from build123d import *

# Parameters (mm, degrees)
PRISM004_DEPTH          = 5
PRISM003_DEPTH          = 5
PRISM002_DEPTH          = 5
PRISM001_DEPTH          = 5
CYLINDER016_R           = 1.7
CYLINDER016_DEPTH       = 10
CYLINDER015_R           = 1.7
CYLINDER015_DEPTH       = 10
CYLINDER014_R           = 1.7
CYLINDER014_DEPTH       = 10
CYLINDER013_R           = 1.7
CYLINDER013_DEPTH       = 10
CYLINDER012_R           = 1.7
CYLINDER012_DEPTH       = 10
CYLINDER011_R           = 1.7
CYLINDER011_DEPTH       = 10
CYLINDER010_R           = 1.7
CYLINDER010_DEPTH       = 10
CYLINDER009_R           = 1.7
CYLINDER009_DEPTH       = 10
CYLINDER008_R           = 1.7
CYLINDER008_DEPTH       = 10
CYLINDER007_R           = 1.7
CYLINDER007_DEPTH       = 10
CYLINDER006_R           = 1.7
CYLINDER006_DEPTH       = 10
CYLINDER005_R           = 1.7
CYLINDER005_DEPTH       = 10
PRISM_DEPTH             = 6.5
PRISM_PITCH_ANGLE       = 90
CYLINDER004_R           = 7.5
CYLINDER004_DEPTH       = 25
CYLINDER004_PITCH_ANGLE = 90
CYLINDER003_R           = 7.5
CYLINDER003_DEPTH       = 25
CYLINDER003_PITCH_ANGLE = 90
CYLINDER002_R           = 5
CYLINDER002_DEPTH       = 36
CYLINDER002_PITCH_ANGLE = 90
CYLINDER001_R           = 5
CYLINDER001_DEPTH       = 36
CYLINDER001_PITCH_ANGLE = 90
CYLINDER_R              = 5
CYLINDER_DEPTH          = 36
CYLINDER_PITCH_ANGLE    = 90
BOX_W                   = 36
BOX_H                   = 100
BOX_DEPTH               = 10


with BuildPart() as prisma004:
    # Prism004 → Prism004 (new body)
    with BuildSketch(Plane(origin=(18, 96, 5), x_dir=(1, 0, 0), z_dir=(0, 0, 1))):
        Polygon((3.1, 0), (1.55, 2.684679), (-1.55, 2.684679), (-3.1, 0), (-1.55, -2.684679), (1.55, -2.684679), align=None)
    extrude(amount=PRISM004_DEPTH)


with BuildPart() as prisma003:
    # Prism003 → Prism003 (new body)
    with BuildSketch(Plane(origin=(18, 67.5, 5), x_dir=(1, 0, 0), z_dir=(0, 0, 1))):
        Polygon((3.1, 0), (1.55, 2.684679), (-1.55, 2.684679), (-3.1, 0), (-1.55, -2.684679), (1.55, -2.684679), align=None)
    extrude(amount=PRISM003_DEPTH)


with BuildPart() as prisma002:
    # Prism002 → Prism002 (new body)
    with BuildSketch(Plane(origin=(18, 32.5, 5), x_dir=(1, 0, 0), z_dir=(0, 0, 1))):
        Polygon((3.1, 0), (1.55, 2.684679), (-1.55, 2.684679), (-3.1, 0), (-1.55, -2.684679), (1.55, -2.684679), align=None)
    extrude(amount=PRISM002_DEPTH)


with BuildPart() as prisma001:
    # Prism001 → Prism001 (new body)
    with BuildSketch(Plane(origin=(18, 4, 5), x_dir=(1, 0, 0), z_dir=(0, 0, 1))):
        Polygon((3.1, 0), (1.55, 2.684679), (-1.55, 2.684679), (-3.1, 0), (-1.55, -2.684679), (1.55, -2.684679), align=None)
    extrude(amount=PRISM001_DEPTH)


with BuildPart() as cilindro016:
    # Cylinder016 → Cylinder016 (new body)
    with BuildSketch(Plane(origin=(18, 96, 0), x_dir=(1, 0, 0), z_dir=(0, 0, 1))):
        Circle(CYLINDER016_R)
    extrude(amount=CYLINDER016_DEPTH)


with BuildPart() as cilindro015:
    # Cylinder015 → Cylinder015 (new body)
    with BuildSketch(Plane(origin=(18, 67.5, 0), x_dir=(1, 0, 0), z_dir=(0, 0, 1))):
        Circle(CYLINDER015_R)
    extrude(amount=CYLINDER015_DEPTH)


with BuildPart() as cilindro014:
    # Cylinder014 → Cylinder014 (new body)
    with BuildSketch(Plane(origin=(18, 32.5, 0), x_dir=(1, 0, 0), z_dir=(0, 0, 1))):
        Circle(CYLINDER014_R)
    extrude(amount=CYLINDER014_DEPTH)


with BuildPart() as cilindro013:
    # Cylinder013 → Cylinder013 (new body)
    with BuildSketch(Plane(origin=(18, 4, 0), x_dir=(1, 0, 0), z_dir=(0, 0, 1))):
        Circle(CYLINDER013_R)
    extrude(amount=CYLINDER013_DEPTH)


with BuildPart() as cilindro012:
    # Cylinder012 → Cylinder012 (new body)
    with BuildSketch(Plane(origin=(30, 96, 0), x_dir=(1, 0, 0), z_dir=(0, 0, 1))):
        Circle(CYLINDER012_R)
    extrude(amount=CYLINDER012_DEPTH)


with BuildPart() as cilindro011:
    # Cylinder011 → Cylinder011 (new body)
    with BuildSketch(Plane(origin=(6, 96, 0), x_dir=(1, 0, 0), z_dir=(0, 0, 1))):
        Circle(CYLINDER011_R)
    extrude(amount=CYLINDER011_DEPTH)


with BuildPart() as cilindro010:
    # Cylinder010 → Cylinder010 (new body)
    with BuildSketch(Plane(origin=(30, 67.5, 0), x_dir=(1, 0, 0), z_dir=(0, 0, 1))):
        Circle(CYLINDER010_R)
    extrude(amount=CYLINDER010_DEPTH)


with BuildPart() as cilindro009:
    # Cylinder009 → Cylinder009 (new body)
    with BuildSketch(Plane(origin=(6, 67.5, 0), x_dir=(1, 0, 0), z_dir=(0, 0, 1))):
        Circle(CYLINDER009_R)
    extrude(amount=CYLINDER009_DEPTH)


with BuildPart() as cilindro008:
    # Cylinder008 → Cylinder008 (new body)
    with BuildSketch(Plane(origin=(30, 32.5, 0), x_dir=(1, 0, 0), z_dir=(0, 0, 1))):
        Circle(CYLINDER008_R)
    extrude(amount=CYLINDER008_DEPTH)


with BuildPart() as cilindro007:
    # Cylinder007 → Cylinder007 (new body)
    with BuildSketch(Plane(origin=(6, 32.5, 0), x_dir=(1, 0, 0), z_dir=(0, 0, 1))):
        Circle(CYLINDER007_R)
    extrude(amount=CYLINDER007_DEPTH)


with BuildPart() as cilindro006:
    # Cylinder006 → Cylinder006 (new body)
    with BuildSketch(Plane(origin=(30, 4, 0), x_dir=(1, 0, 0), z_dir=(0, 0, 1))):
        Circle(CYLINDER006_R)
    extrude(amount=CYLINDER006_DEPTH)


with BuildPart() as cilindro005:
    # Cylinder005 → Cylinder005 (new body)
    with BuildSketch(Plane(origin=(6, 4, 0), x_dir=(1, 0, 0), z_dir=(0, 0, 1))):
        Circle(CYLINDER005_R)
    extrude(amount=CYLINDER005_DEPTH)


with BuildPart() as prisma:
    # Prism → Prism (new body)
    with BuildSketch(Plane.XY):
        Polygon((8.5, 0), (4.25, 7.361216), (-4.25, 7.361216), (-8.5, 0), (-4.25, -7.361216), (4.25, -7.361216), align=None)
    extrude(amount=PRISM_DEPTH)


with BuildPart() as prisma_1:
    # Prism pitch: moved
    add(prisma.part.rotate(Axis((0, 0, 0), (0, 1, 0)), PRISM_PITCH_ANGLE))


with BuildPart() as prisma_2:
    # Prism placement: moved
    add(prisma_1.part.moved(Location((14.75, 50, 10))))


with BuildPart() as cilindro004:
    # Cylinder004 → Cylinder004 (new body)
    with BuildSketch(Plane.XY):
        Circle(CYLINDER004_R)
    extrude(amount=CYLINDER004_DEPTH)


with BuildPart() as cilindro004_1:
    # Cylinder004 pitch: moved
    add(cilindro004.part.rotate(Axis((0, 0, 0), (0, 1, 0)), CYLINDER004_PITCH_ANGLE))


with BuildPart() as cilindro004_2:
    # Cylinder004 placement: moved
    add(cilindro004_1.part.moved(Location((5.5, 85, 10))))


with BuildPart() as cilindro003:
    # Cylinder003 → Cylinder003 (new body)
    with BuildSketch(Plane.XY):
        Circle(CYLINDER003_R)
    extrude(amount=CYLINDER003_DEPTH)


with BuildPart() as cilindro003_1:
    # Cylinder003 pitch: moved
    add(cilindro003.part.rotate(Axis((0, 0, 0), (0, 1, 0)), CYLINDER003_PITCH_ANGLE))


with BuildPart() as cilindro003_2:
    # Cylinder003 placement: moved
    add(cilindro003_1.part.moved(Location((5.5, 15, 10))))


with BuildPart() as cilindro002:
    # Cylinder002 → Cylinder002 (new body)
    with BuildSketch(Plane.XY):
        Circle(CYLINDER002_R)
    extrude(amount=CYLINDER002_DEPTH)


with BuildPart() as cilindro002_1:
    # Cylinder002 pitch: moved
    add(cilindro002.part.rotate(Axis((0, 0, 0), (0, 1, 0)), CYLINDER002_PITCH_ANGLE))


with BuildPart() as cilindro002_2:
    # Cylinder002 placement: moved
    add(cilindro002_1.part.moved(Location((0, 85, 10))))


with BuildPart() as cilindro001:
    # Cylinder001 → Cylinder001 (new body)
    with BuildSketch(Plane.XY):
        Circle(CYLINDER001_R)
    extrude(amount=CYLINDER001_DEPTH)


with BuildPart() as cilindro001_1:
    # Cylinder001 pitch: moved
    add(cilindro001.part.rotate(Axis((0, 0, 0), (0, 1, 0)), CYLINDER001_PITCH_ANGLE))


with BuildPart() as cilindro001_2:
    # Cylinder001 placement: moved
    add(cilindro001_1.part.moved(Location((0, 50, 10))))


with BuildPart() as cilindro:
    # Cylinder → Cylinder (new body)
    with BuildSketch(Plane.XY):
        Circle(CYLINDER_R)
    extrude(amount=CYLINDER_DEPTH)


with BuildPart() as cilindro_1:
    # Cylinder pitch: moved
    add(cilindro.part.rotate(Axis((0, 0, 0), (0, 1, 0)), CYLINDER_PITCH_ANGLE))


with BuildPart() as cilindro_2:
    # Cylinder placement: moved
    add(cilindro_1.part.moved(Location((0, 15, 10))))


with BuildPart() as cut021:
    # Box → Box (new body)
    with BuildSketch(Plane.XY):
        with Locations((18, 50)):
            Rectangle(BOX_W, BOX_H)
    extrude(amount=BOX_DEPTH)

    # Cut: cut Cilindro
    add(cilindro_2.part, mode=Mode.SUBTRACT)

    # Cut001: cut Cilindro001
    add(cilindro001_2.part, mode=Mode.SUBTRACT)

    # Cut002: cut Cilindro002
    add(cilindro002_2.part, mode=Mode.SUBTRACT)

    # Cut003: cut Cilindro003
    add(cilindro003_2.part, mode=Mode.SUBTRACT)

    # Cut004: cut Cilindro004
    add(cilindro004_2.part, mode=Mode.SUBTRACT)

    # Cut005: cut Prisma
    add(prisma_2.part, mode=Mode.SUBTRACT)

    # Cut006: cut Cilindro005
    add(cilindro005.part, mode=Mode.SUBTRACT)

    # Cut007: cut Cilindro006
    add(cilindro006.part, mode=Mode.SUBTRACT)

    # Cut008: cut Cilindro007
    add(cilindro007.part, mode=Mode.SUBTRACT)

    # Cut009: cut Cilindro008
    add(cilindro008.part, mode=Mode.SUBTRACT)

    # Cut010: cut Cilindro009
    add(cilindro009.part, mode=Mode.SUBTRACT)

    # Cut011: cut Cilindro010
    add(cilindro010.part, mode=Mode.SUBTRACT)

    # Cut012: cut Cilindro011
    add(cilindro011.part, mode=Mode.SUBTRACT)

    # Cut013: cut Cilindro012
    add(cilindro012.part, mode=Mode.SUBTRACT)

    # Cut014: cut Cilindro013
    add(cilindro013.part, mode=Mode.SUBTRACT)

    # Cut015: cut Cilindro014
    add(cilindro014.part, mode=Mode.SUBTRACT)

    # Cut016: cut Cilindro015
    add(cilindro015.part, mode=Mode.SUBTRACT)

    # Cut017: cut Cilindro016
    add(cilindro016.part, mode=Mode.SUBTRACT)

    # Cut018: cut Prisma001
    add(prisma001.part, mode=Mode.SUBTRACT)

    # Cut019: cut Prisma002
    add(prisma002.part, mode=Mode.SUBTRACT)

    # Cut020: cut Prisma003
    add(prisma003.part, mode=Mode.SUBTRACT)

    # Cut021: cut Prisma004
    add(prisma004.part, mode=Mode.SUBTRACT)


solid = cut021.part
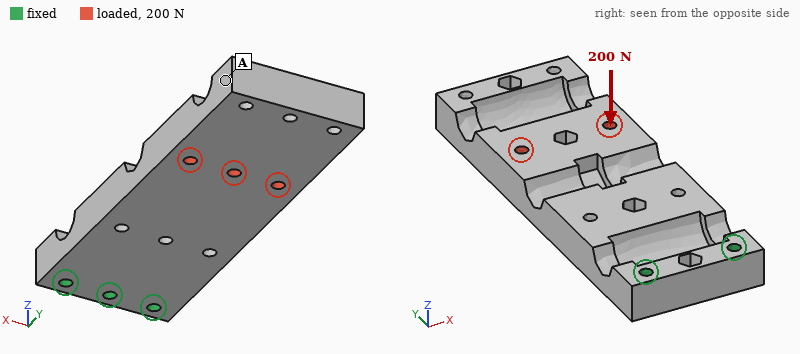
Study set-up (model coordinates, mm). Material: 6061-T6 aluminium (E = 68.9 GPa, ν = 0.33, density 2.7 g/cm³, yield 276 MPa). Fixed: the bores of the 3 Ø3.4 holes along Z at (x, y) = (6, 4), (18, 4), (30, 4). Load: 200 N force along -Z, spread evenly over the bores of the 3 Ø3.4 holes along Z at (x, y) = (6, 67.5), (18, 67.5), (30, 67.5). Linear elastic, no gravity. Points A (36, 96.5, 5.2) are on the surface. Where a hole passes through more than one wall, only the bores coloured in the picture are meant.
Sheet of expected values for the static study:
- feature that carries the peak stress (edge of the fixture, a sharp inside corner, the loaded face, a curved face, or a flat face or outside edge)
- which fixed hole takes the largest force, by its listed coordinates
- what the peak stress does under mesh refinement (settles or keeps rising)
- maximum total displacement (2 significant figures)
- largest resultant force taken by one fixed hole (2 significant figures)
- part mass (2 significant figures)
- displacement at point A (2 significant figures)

a sharp inside corner
(18, 4)
keeps rising
0.78 mm
700 N
74 g
0.75 mm
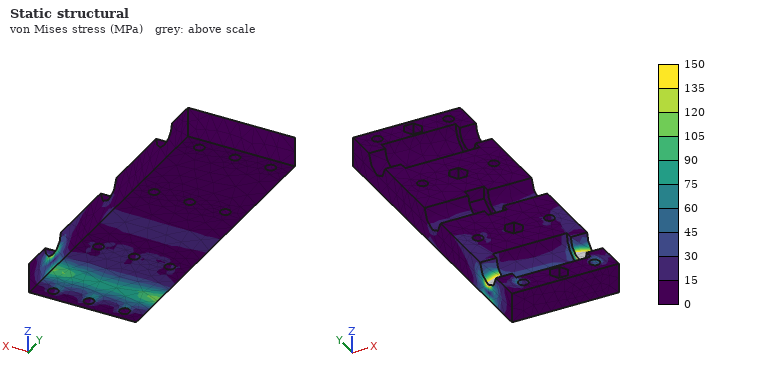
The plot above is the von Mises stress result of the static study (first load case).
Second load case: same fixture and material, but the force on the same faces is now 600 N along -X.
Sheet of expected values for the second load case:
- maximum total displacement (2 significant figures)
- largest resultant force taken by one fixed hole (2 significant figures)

79 µm
1.4 kN
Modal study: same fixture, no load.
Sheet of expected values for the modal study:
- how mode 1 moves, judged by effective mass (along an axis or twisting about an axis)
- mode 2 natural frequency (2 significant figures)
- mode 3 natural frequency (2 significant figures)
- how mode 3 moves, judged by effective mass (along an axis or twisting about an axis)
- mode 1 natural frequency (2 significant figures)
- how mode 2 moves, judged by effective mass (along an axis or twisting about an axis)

along Z
2400 Hz
3200 Hz
along Z
440 Hz
along X
